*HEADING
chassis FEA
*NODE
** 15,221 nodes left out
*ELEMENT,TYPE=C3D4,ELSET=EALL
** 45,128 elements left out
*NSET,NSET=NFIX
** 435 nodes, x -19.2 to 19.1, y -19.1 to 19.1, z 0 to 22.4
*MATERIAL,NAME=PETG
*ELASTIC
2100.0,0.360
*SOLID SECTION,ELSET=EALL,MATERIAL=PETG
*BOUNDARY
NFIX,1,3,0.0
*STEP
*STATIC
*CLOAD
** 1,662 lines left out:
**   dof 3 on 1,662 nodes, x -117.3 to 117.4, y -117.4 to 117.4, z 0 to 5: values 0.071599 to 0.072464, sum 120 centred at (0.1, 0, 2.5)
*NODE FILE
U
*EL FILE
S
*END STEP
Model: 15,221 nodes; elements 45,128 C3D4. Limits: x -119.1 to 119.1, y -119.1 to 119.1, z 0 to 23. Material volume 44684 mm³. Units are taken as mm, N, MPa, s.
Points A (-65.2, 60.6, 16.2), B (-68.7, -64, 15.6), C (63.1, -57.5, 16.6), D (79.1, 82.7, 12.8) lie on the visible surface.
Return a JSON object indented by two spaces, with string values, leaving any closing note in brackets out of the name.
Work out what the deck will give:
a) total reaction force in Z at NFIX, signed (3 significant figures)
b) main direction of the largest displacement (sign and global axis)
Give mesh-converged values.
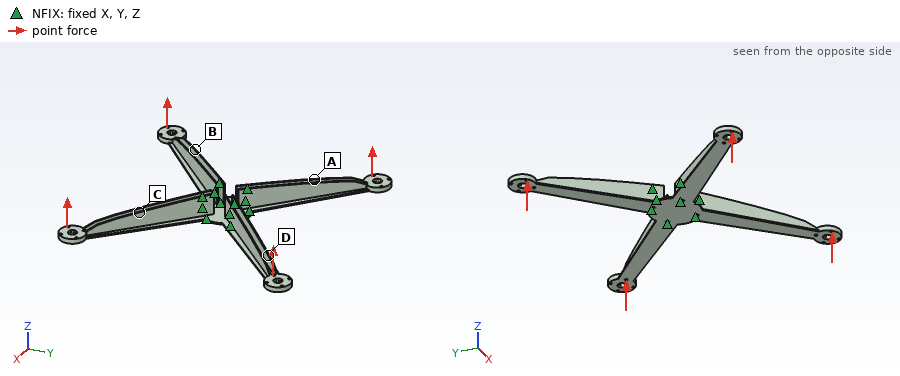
{
  "total reaction force in Z at NFIX, signed": "-120 N",
  "main direction of the largest displacement": "+Z"
}
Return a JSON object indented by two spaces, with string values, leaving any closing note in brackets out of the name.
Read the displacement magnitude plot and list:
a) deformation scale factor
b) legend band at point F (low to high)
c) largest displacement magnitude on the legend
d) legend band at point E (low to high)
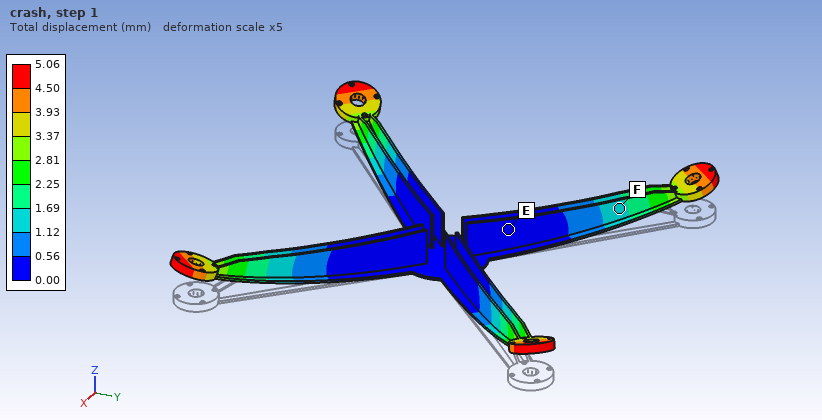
{
  "deformation scale factor": "5",
  "legend band at point F": "1.12 to 1.69 mm",
  "largest displacement magnitude on the legend": "5.06 mm",
  "legend band at point E": "0.00 to 0.56 mm"
}
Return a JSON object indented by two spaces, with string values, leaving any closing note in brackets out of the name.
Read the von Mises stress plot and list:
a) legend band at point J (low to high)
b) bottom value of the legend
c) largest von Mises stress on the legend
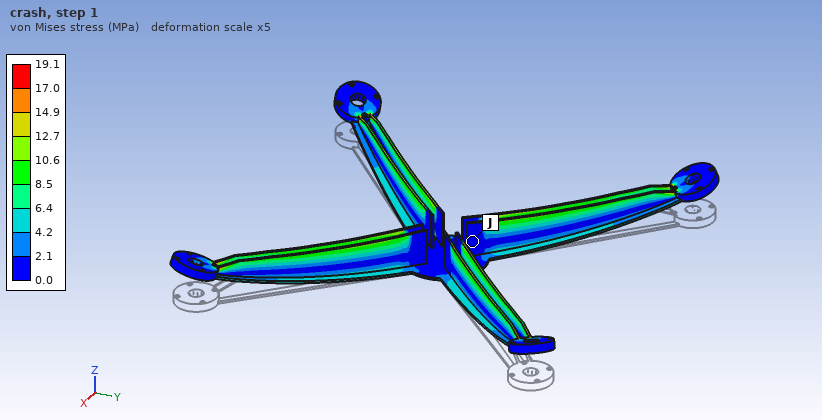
{
  "legend band at point J": "0.0 to 2.1 MPa",
  "bottom value of the legend": "0.0 MPa",
  "largest von Mises stress on the legend": "19.1 MPa"
}
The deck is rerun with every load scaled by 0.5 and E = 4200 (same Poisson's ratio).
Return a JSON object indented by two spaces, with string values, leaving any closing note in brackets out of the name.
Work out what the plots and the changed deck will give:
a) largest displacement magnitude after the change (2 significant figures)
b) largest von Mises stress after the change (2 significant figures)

{
  "largest displacement magnitude after the change": "1.3 mm",
  "largest von Mises stress after the change": "9.6 MPa"
}
